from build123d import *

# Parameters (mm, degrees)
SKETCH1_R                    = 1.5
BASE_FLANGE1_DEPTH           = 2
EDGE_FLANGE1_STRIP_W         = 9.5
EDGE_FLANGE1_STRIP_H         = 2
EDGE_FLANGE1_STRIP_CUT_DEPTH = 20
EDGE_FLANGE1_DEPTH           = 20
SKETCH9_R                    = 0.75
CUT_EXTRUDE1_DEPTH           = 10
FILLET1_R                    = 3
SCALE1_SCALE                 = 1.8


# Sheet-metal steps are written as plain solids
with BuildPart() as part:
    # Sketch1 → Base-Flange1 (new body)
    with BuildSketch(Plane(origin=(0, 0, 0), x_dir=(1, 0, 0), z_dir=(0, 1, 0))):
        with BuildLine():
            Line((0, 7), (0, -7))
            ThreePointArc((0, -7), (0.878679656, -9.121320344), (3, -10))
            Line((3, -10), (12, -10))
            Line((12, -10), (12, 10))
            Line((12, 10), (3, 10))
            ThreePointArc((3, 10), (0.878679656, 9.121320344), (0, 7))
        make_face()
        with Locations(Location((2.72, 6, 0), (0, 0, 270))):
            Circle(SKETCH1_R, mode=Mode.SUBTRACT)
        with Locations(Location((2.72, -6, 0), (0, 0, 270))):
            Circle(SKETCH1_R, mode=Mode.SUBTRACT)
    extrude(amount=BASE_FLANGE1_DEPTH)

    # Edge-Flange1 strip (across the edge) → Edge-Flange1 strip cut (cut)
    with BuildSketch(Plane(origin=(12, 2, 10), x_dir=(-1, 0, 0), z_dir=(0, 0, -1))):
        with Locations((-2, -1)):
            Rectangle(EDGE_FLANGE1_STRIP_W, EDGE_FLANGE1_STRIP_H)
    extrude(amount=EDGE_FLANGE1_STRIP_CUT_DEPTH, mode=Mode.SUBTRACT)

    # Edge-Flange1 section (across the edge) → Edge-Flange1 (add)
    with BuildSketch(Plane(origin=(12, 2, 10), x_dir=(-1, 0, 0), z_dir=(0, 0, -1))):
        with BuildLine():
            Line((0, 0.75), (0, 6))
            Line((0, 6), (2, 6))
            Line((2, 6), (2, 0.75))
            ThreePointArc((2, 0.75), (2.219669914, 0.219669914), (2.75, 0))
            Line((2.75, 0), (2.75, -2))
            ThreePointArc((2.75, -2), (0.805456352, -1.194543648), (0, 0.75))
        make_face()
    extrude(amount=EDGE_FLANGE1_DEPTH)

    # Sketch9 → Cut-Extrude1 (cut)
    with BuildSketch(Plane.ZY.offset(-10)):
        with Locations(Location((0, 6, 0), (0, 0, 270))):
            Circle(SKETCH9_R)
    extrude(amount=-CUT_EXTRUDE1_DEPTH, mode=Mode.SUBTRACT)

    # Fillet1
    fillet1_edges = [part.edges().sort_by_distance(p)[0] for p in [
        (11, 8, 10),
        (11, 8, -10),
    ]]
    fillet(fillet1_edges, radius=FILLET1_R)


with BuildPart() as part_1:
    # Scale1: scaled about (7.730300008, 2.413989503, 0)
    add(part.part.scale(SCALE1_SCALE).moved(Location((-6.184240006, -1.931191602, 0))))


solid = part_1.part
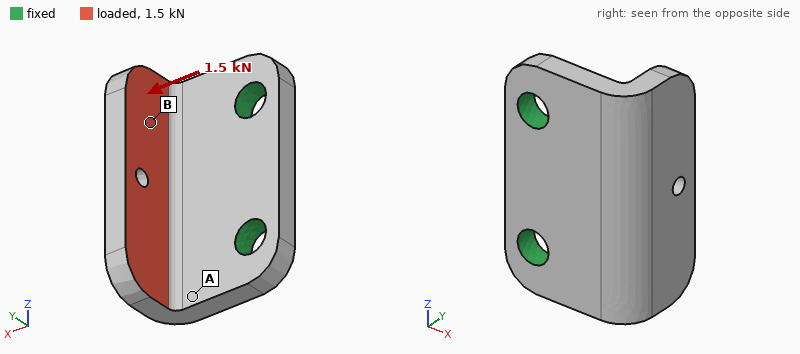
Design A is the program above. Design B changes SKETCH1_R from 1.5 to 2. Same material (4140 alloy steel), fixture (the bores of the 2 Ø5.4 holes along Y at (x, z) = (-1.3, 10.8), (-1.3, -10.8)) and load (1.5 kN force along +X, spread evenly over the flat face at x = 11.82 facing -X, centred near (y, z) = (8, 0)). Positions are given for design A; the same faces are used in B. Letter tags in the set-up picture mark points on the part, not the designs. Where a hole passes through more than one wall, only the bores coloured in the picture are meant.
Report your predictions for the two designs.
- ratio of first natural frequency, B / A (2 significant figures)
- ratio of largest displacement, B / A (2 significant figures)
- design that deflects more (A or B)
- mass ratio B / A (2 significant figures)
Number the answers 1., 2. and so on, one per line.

1. 1.1
2. 0.90
3. A
4. 0.97
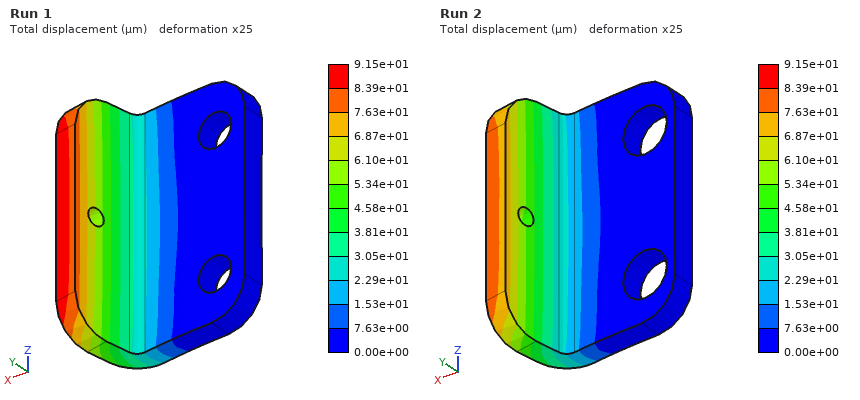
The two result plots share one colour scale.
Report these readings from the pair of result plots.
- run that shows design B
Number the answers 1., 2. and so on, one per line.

1. Run 2
